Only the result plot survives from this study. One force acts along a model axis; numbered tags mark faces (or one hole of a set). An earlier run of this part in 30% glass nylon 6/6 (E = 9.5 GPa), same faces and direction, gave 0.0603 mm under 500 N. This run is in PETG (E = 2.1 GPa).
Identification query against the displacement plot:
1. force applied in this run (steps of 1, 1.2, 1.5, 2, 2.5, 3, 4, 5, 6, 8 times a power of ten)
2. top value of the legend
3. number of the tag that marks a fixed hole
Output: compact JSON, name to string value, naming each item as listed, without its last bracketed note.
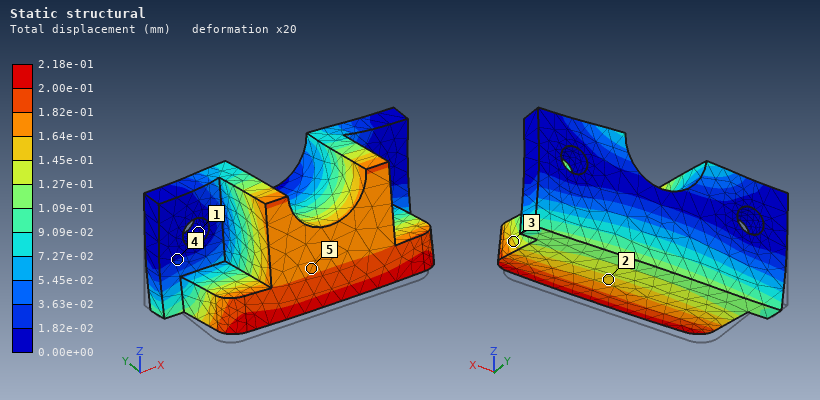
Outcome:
{"force applied in this run": "400 N", "top value of the legend": "2.18e-01 mm", "number of the tag that marks a fixed hole": "1"}
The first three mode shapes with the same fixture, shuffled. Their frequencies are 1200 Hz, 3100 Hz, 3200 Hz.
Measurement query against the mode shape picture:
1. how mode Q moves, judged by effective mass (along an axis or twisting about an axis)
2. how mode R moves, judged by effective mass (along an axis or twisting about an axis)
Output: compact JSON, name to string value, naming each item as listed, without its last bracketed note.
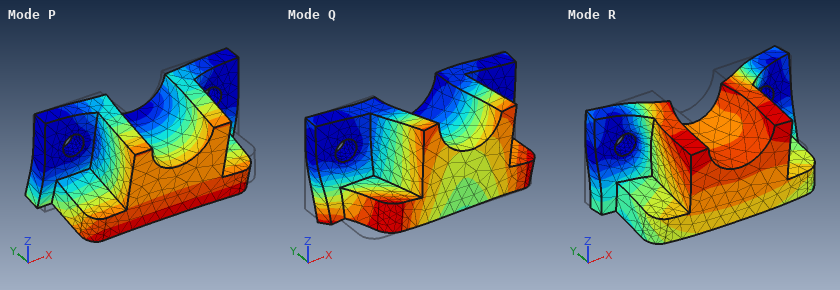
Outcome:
{"how mode Q moves, judged by effective mass": "along X", "how mode R moves, judged by effective mass": "along Y"}
